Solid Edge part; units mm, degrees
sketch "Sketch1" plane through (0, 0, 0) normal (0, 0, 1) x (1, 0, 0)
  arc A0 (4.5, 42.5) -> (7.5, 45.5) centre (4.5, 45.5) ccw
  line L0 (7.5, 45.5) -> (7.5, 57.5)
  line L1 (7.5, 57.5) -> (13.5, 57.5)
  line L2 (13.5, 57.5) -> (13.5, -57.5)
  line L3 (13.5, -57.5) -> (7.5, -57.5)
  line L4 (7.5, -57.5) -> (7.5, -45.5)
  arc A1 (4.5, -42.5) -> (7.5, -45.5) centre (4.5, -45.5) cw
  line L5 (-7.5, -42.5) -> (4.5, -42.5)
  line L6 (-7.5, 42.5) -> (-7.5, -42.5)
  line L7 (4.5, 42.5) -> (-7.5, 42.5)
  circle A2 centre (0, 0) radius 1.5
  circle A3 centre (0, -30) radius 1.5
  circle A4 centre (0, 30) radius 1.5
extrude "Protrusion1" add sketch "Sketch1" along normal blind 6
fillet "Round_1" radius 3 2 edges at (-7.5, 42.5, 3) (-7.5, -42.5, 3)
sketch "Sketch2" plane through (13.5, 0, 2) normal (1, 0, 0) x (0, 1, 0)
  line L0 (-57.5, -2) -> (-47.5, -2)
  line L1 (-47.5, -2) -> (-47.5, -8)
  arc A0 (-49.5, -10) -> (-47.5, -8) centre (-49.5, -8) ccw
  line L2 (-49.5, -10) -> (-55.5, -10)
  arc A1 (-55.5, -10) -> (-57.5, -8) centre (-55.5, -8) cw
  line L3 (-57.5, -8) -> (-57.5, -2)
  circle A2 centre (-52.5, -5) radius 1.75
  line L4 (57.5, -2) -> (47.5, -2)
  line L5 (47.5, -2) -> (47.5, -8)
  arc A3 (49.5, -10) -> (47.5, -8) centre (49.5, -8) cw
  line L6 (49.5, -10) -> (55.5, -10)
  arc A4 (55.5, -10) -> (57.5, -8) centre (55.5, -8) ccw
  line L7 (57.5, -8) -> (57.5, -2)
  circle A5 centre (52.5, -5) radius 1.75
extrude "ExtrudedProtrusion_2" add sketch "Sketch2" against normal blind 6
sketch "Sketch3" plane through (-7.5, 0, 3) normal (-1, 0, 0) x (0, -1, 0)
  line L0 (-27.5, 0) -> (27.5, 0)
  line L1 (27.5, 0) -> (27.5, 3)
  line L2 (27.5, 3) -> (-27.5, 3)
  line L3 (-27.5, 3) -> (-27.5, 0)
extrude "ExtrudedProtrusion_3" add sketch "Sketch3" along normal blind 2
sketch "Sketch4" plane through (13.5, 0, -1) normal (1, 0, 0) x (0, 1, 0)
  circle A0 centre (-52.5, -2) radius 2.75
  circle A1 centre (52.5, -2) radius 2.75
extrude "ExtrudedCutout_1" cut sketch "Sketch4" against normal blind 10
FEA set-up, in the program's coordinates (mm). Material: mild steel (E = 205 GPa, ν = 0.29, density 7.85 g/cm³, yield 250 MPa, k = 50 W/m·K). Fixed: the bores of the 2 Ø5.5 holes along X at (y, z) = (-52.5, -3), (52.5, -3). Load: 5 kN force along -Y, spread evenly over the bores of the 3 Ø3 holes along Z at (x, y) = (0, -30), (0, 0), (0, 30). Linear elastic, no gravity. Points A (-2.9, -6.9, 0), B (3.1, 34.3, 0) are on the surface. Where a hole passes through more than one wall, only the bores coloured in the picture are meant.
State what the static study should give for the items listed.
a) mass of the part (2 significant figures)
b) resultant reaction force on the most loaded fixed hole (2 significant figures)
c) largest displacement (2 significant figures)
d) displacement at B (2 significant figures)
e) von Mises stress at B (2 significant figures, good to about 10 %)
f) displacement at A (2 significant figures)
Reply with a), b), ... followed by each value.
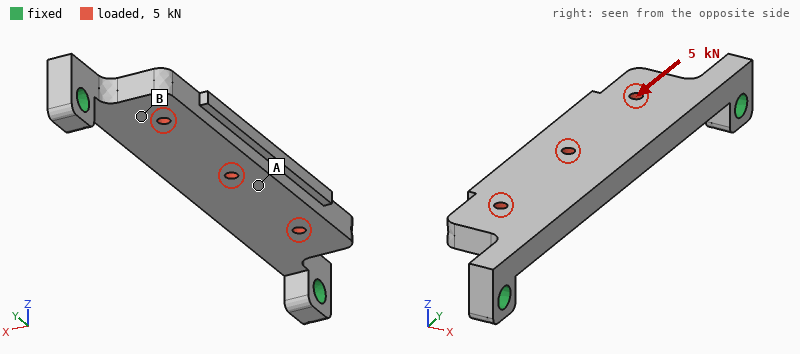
a) 99 g
b) 2.6 kN
c) 14 µm
d) 11 µm
e) 37 MPa
f) 11 µm
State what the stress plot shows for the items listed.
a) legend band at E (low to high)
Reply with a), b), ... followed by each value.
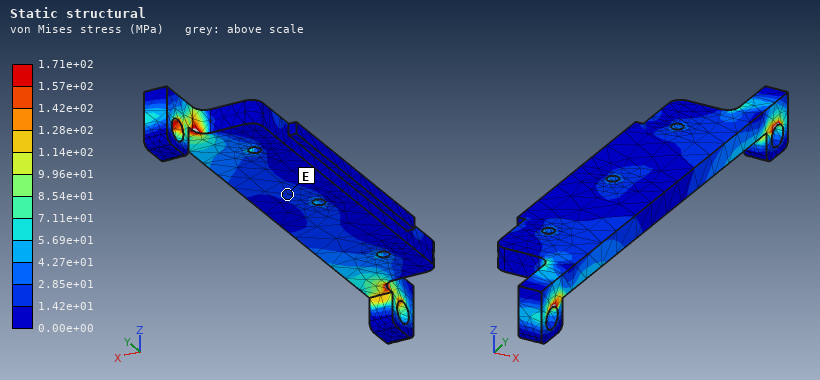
a) 1.42e+01 to 2.85e+01 MPa
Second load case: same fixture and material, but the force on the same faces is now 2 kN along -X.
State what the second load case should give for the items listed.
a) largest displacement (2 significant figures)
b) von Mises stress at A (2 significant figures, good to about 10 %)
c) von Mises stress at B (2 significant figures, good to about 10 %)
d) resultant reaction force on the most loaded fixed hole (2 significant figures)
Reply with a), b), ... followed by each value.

a) 32 µm
b) 27 MPa
c) 26 MPa
d) 1.4 kN
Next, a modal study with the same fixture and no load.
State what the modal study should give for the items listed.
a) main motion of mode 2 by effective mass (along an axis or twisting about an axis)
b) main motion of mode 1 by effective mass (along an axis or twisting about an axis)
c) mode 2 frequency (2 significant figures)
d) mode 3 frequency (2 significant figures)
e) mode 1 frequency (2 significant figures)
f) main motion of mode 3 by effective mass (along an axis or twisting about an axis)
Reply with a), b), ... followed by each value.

a) twisting about Y
b) along Z
c) 4400 Hz
d) 5200 Hz
e) 1900 Hz
f) along X
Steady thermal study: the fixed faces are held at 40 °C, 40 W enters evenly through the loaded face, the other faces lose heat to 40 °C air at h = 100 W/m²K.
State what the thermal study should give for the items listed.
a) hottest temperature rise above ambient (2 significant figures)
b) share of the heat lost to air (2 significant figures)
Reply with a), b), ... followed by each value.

a) 73 K
b) 70 %
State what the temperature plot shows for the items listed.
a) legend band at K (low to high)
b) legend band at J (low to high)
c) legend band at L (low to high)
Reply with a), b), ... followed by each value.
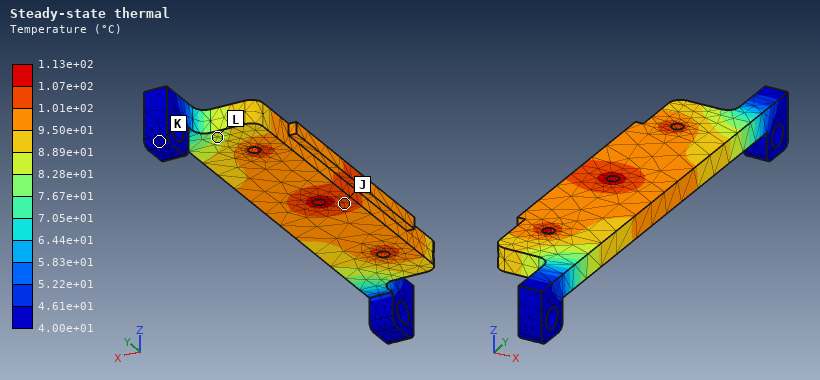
a) 4.00e+01 to 4.61e+01 °C
b) 1.01e+02 to 1.07e+02 °C
c) 8.28e+01 to 8.89e+01 °C
